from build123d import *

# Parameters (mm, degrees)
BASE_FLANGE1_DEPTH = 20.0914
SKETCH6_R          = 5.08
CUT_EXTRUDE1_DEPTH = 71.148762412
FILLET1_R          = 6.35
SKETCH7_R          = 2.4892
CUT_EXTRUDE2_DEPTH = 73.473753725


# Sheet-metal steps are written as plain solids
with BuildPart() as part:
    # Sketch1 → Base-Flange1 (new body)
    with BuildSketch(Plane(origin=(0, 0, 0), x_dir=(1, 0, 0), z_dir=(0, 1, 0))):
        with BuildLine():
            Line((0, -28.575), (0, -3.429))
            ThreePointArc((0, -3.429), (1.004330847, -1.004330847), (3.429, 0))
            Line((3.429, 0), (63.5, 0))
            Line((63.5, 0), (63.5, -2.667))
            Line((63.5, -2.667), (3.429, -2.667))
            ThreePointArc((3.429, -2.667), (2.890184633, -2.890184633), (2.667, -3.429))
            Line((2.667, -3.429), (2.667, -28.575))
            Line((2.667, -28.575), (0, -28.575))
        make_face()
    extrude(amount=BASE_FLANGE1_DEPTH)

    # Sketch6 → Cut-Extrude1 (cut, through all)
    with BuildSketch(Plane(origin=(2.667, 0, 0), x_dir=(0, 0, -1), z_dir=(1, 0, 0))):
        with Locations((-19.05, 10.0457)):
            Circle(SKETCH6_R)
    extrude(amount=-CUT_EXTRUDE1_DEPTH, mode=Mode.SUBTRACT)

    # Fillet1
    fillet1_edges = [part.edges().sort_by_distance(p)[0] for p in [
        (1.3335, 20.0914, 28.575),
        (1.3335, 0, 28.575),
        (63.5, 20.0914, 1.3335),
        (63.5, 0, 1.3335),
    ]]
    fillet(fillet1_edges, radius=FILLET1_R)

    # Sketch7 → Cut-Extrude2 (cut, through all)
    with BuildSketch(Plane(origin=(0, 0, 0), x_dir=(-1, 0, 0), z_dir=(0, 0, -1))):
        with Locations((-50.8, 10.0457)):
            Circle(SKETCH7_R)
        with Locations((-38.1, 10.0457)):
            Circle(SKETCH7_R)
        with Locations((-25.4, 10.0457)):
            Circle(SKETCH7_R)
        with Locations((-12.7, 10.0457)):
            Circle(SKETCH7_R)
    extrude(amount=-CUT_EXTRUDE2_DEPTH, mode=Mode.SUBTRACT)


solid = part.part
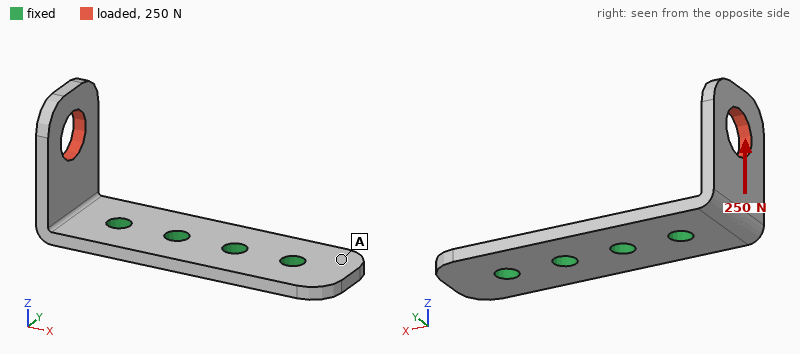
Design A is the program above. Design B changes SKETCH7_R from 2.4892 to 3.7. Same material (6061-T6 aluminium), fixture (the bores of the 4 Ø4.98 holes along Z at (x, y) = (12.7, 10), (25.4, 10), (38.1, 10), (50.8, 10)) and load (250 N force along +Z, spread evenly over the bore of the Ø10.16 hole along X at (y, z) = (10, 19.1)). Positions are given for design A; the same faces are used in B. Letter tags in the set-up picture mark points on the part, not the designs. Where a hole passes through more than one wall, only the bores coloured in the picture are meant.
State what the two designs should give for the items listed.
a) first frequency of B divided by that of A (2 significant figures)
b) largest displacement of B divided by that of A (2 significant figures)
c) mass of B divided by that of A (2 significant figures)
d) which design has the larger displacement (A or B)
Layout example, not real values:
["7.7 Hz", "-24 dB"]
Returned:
["1.1", "0.74", "0.94", "A"]
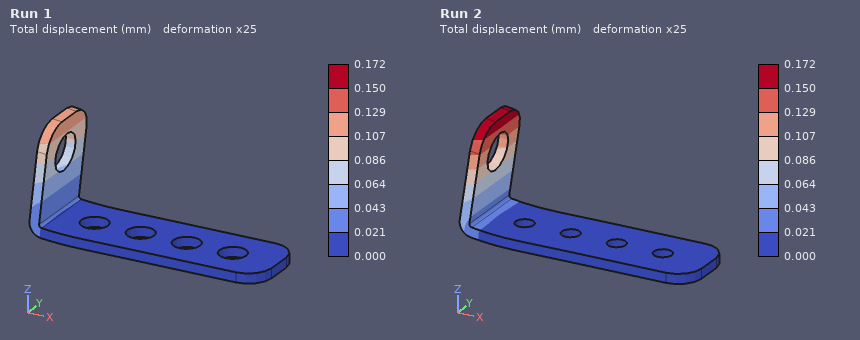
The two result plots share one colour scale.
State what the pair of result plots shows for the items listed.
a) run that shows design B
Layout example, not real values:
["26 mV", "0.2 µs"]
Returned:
["Run 1"]
